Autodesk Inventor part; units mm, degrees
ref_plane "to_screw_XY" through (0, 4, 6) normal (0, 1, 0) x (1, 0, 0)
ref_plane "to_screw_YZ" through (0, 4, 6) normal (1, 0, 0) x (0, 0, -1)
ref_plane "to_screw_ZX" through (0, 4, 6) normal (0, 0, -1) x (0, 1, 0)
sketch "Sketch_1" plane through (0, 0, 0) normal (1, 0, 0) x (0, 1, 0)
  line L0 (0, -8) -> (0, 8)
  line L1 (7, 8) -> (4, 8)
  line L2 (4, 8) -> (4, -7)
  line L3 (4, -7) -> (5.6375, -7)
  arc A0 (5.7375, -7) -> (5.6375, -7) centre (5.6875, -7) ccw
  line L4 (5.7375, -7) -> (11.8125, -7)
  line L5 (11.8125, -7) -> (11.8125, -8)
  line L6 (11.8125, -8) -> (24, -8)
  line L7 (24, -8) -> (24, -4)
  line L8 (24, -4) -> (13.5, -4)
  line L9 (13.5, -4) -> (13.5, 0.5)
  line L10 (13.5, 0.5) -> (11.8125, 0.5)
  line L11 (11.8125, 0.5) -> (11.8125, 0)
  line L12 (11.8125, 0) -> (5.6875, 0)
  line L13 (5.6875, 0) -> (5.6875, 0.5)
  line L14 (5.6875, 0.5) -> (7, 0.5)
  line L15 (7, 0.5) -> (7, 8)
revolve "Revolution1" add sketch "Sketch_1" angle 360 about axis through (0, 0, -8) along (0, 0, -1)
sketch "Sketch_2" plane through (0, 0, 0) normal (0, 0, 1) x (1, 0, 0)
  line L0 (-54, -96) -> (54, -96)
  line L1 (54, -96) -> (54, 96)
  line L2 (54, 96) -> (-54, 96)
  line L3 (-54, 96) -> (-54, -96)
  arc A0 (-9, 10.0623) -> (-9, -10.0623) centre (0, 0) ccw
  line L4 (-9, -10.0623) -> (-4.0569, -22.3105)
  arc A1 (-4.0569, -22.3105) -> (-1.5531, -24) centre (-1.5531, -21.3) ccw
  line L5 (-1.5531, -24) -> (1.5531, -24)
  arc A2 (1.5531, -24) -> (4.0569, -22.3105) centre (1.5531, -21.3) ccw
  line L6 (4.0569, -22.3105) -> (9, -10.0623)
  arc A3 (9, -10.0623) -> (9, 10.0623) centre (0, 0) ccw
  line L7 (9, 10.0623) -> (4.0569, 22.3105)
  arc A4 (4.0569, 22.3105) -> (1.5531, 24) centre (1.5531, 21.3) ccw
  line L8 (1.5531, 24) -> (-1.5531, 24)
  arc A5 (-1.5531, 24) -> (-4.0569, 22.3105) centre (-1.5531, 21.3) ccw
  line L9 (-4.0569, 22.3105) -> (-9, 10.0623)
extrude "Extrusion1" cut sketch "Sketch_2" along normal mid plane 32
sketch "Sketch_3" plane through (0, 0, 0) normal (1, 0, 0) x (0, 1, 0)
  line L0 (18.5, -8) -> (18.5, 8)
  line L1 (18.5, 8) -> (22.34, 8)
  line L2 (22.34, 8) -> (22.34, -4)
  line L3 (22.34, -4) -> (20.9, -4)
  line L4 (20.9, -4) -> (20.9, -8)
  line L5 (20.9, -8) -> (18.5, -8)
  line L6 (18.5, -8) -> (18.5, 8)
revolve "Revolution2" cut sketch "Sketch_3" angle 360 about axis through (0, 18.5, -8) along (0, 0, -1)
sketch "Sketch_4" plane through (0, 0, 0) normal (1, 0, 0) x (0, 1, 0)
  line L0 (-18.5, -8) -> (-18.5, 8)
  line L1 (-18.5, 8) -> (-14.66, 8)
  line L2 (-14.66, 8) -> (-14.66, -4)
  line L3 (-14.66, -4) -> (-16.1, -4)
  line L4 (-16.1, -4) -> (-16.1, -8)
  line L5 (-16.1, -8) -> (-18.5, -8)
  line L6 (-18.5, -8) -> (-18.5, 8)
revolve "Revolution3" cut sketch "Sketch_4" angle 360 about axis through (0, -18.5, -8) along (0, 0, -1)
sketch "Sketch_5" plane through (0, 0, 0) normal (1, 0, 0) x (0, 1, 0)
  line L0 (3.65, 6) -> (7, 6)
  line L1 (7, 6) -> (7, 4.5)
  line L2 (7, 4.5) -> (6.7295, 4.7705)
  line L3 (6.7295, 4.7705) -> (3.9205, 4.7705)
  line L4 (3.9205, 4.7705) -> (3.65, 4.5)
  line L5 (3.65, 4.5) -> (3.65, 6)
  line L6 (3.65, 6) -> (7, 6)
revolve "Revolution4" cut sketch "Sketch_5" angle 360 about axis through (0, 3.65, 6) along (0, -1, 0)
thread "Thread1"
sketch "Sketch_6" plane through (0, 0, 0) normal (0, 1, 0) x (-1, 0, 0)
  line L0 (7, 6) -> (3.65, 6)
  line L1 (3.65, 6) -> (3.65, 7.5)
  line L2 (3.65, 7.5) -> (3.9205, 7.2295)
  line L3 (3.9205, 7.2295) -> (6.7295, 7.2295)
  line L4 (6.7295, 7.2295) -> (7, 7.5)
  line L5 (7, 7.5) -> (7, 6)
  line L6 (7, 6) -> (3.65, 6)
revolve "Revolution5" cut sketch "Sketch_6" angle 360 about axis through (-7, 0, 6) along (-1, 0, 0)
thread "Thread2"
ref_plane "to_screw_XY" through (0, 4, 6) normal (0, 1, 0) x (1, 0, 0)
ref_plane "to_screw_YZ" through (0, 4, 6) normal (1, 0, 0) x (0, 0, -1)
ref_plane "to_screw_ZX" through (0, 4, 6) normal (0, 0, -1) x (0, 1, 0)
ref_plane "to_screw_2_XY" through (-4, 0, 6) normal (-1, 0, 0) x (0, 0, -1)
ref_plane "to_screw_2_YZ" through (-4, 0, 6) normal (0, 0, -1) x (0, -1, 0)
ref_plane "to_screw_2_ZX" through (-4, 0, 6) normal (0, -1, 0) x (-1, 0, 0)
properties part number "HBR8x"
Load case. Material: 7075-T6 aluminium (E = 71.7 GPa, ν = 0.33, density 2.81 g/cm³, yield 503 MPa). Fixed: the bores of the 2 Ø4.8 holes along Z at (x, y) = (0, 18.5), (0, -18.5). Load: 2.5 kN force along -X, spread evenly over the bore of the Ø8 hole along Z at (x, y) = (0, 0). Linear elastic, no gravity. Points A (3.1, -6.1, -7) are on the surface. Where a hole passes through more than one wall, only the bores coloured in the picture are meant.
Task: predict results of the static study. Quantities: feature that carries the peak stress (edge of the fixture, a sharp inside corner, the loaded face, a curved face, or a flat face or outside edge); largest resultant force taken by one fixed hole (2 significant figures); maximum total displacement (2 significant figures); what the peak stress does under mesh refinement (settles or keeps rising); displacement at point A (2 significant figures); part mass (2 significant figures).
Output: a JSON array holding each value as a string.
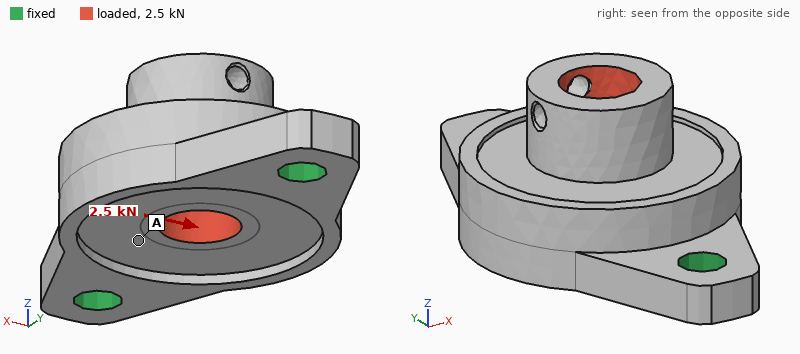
["edge of the fixture", "1.3 kN", "0.11 mm", "keeps rising", "0.018 mm", "16 g"]
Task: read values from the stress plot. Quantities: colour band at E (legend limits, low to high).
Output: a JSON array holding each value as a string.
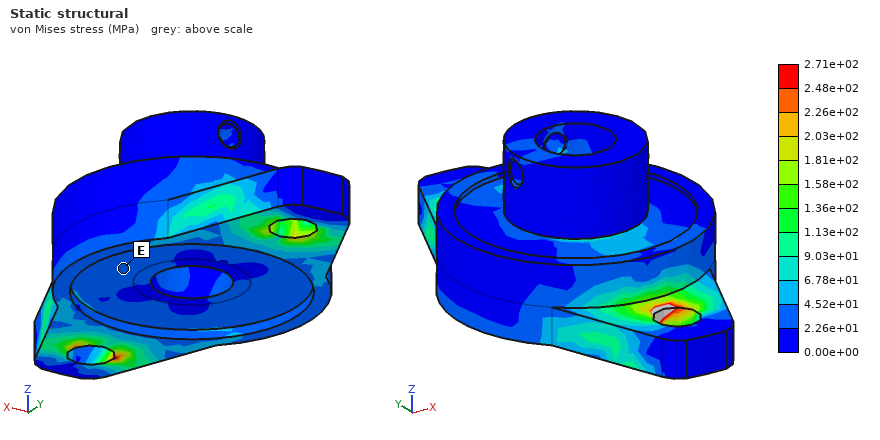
["2.26e+01 to 4.52e+01 MPa"]
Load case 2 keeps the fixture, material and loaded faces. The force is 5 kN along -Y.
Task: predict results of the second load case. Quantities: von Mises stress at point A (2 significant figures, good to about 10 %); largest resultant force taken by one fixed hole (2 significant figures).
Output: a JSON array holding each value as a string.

["20 MPa", "2.7 kN"]
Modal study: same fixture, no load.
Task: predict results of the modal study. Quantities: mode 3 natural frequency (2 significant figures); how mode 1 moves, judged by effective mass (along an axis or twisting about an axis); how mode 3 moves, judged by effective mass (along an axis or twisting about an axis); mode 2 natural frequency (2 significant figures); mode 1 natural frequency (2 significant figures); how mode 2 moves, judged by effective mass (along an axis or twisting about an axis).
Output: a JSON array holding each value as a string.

["26 kHz", "along X", "along X", "14 kHz", "8400 Hz", "along Z"]
